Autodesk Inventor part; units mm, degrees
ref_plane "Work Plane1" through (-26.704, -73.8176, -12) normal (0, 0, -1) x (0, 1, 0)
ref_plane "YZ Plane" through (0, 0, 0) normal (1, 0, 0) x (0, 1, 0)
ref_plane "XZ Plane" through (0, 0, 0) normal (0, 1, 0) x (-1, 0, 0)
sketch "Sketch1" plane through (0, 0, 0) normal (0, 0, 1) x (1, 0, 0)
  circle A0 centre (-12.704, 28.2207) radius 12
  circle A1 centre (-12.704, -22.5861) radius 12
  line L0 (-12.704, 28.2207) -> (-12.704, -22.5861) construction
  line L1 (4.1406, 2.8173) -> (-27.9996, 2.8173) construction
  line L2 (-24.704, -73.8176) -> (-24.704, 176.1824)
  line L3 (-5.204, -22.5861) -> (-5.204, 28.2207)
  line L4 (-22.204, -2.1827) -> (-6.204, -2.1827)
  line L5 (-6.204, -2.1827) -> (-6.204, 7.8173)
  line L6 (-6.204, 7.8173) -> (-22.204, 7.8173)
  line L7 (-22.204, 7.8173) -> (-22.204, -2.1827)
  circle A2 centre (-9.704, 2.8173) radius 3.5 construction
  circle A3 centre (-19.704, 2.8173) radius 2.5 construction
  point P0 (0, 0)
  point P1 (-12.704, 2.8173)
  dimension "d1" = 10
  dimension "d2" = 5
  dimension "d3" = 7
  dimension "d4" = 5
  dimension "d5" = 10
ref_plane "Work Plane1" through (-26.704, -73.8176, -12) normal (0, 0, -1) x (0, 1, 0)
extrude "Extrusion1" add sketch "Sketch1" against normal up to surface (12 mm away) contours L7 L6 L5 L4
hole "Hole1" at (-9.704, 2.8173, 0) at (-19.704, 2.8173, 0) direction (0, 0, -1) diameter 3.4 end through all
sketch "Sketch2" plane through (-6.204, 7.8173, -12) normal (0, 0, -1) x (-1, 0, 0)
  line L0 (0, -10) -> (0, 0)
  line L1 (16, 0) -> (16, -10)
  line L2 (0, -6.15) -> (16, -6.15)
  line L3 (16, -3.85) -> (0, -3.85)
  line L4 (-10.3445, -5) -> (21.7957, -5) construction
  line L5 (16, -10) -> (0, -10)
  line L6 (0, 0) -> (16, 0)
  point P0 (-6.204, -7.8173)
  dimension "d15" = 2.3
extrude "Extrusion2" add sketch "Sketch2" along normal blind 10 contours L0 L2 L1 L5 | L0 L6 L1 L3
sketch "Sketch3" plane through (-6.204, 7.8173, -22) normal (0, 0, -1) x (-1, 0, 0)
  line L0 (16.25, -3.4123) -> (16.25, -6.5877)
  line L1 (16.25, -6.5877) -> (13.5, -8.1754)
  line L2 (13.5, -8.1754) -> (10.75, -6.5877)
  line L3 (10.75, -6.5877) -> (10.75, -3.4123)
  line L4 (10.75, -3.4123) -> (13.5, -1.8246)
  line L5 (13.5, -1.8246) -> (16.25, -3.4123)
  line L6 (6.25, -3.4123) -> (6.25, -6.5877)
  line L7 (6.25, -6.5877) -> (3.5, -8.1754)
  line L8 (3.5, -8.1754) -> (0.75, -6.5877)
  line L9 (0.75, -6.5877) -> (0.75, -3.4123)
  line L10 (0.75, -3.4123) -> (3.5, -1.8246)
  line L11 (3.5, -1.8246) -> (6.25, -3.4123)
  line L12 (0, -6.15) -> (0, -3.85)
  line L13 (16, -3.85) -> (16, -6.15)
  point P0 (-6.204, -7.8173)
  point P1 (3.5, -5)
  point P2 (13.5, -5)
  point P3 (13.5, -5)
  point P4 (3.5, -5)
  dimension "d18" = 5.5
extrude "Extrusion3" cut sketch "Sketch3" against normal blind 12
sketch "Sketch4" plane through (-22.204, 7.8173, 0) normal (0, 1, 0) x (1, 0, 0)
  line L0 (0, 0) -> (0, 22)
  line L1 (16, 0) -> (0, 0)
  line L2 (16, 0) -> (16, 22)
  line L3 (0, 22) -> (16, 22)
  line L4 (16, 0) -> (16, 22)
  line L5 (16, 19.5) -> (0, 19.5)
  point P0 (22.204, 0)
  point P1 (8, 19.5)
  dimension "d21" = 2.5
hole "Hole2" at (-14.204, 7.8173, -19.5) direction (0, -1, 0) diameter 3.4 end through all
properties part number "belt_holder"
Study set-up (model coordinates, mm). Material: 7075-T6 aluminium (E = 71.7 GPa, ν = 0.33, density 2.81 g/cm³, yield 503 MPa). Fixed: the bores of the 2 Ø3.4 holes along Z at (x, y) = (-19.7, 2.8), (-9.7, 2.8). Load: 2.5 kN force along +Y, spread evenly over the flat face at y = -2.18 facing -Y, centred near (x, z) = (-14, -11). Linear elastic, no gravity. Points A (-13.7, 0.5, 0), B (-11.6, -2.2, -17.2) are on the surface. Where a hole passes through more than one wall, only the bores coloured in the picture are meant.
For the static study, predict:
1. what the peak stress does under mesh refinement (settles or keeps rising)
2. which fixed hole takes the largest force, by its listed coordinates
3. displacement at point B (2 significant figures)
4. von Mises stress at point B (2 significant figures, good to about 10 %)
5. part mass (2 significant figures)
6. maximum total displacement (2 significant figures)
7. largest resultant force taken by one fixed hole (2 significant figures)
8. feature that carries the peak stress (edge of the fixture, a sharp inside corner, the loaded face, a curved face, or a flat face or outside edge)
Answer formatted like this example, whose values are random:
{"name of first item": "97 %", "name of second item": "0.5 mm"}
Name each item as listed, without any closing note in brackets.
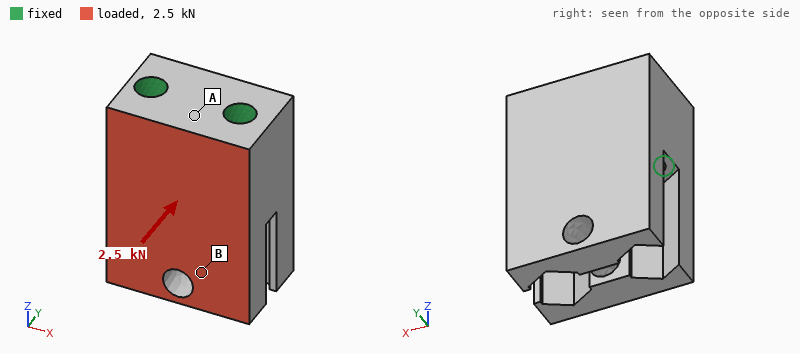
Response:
{"what the peak stress does under mesh refinement": "keeps rising", "which fixed hole takes the largest force, by its listed coordinates": "(-9.7, 2.8)", "displacement at point B": "0.057 mm", "von Mises stress at point B": "46 MPa", "part mass": "7.1 g", "maximum total displacement": "0.11 mm", "largest resultant force taken by one fixed hole": "1.4 kN", "feature that carries the peak stress": "a sharp inside corner"}
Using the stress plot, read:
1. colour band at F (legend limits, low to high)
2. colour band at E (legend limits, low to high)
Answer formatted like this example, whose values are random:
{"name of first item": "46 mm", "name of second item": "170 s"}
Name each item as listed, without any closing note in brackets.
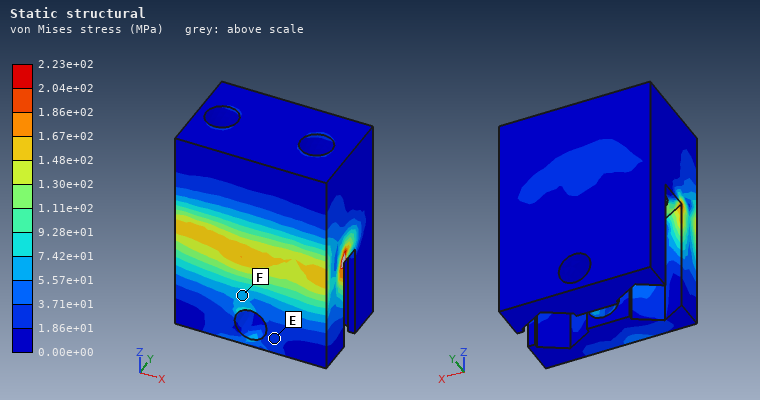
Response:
{"colour band at F": "5.57e+01 to 7.42e+01 MPa", "colour band at E": "1.86e+01 to 3.71e+01 MPa"}
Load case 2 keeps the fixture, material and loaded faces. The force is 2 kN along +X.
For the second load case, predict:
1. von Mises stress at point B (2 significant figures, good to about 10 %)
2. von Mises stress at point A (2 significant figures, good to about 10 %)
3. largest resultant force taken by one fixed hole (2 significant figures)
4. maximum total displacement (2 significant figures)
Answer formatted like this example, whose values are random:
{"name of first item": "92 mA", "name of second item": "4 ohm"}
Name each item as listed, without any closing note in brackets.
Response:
{"von Mises stress at point B": "38 MPa", "von Mises stress at point A": "8.6 MPa", "largest resultant force taken by one fixed hole": "1.4 kN", "maximum total displacement": "29 µm"}
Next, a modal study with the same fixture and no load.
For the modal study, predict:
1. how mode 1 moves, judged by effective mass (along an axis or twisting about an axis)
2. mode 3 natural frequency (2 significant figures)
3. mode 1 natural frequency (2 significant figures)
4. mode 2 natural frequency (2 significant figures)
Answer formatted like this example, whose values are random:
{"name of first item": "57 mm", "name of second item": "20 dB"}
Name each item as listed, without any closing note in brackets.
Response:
{"how mode 1 moves, judged by effective mass": "along Y", "mode 3 natural frequency": "27 kHz", "mode 1 natural frequency": "18 kHz", "mode 2 natural frequency": "19 kHz"}
